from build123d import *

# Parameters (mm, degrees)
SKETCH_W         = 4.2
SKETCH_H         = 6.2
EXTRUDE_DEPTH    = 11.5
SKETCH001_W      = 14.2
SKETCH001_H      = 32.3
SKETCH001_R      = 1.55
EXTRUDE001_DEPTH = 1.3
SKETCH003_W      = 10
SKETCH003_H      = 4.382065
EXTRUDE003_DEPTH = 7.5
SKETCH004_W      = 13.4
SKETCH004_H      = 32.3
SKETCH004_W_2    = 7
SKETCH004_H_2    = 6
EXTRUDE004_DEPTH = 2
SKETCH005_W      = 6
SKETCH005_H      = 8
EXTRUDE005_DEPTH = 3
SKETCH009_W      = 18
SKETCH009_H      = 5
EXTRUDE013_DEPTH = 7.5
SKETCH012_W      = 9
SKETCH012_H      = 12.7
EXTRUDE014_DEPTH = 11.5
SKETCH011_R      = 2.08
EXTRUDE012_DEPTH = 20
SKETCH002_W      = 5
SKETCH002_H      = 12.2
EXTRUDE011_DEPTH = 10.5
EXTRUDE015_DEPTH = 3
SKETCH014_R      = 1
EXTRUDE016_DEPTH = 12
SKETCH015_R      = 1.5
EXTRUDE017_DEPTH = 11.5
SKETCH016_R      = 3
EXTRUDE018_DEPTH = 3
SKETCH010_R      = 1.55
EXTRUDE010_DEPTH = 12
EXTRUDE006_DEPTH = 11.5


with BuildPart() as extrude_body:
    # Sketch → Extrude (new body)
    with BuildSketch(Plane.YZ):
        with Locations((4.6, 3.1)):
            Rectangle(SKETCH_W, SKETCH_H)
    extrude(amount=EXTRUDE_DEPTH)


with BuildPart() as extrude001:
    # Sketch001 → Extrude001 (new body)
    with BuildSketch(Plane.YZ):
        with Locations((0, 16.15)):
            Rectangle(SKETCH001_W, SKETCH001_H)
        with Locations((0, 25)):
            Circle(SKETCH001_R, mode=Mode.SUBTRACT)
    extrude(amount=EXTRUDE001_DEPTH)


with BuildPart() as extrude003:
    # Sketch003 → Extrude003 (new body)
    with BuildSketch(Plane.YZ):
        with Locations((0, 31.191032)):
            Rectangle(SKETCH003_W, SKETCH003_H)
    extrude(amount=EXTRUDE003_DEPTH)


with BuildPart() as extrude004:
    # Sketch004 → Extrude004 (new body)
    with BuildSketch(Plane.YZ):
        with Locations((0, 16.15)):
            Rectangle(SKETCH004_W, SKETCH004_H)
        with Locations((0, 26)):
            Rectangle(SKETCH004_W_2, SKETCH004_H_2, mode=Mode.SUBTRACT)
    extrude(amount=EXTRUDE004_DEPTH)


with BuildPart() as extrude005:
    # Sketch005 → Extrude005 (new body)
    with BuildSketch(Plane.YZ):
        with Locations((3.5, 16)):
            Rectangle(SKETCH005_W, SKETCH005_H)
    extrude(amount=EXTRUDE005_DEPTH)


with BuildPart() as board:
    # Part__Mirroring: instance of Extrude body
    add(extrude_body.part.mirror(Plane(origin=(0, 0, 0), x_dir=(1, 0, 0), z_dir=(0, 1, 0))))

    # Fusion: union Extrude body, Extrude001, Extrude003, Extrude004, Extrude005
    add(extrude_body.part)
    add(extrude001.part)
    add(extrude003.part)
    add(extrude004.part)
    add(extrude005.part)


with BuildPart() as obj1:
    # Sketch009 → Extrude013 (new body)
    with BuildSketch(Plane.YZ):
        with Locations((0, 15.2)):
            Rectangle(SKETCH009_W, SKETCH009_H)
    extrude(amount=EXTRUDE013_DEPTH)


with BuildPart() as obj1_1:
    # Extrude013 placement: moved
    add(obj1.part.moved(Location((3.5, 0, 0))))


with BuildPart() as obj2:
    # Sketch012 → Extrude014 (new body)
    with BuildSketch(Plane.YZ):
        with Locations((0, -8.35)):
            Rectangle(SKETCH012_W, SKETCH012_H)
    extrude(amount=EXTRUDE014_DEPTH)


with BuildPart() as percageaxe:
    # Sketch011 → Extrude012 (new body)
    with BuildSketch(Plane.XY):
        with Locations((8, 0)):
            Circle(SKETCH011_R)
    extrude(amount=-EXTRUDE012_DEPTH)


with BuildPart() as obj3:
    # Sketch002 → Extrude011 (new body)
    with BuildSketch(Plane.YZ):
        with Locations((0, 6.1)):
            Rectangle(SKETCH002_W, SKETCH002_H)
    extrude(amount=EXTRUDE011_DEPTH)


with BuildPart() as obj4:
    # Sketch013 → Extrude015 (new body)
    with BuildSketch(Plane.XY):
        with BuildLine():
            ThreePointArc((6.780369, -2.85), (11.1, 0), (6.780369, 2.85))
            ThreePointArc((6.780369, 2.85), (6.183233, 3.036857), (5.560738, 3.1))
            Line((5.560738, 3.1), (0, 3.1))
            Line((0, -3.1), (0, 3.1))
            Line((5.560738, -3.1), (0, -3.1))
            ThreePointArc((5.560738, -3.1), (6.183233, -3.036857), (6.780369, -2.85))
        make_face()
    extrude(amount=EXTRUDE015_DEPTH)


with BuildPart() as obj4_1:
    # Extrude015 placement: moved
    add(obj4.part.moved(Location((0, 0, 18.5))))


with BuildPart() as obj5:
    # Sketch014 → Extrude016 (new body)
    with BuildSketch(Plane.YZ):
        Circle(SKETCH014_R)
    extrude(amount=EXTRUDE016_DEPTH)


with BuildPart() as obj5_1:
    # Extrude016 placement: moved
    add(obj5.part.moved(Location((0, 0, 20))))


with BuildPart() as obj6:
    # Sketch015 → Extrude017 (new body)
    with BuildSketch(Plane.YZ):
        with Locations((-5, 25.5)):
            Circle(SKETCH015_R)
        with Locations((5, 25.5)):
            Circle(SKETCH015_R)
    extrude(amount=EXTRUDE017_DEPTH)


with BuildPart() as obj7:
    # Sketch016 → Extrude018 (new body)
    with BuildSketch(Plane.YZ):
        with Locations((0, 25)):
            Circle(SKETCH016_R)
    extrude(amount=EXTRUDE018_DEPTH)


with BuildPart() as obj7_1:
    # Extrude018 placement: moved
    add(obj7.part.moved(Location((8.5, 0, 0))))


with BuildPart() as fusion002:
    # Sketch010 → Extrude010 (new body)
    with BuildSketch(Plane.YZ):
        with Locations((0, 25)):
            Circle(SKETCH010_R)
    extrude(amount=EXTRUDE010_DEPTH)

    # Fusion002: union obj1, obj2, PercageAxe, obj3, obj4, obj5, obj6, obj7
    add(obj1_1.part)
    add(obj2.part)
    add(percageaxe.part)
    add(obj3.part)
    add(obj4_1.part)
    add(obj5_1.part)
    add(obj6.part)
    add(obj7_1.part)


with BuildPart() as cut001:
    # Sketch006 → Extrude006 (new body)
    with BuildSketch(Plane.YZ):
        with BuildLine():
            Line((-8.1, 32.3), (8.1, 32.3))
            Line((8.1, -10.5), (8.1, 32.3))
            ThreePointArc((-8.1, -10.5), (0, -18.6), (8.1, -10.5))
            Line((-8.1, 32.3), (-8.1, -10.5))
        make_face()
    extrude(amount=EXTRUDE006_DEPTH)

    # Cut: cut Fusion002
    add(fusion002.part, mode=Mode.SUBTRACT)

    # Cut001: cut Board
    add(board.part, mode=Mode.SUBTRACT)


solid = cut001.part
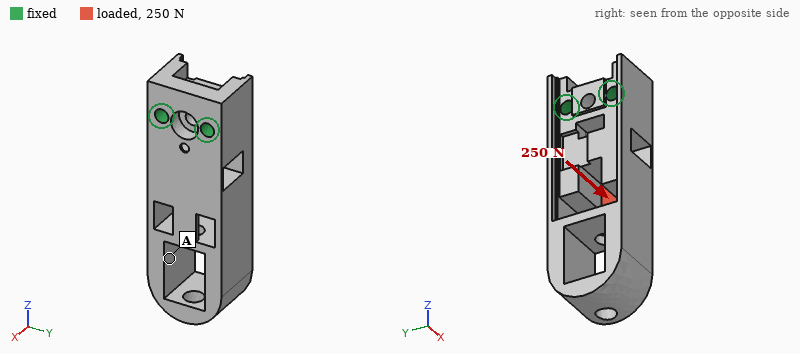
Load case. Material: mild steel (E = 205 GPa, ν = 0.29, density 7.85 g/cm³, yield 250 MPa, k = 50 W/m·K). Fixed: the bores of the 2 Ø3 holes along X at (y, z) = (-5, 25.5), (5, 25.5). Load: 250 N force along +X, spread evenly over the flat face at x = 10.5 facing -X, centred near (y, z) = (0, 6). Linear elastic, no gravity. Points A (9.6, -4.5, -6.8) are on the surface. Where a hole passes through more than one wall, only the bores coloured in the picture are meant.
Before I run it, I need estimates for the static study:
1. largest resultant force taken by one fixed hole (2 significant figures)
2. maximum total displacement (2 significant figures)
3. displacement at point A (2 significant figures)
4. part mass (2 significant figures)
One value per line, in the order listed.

130 N
20 µm
15 µm
36 g
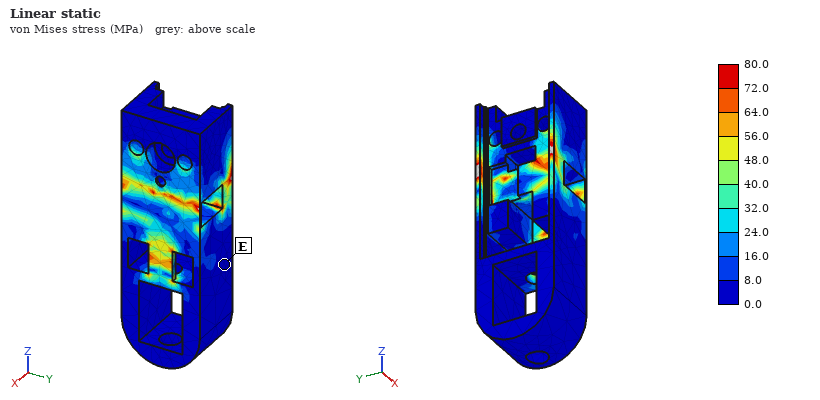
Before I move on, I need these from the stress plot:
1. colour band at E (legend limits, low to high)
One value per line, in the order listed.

0.0 to 8.0 MPa
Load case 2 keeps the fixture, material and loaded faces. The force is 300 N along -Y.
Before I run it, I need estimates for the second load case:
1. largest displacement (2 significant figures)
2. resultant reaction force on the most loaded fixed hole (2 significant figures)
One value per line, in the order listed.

15 µm
430 N
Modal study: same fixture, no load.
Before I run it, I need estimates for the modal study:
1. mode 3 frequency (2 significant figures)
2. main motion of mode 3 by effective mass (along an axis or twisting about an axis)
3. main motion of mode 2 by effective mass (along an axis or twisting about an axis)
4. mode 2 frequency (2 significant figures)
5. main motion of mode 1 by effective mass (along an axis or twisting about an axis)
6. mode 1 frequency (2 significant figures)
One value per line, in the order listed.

8200 Hz
twisting about Z
along Y
3800 Hz
along X
3400 Hz
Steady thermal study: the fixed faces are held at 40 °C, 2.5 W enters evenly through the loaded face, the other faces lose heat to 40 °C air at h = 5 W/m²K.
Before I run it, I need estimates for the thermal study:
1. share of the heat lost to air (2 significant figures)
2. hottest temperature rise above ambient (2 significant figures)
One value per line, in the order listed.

9.5 %
27 K
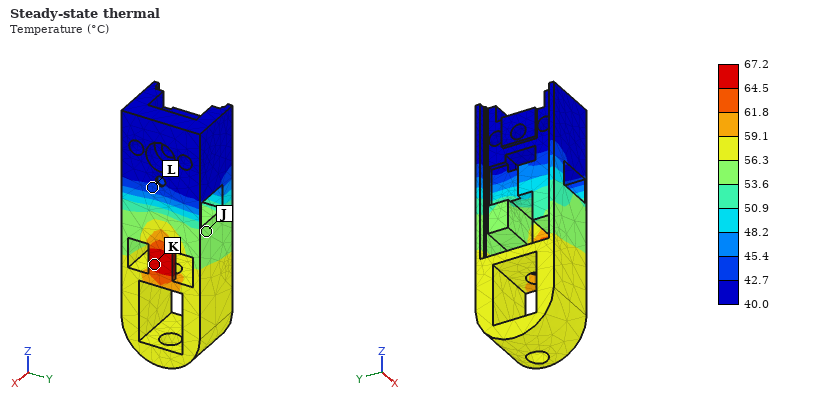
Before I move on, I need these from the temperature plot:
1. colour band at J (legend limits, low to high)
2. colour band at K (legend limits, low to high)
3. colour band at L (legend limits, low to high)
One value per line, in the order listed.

53.6 to 56.3 °C
64.5 to 67.2 °C
42.7 to 45.4 °C
